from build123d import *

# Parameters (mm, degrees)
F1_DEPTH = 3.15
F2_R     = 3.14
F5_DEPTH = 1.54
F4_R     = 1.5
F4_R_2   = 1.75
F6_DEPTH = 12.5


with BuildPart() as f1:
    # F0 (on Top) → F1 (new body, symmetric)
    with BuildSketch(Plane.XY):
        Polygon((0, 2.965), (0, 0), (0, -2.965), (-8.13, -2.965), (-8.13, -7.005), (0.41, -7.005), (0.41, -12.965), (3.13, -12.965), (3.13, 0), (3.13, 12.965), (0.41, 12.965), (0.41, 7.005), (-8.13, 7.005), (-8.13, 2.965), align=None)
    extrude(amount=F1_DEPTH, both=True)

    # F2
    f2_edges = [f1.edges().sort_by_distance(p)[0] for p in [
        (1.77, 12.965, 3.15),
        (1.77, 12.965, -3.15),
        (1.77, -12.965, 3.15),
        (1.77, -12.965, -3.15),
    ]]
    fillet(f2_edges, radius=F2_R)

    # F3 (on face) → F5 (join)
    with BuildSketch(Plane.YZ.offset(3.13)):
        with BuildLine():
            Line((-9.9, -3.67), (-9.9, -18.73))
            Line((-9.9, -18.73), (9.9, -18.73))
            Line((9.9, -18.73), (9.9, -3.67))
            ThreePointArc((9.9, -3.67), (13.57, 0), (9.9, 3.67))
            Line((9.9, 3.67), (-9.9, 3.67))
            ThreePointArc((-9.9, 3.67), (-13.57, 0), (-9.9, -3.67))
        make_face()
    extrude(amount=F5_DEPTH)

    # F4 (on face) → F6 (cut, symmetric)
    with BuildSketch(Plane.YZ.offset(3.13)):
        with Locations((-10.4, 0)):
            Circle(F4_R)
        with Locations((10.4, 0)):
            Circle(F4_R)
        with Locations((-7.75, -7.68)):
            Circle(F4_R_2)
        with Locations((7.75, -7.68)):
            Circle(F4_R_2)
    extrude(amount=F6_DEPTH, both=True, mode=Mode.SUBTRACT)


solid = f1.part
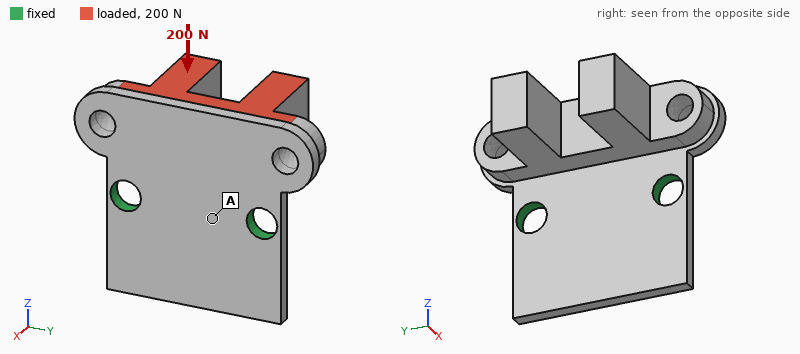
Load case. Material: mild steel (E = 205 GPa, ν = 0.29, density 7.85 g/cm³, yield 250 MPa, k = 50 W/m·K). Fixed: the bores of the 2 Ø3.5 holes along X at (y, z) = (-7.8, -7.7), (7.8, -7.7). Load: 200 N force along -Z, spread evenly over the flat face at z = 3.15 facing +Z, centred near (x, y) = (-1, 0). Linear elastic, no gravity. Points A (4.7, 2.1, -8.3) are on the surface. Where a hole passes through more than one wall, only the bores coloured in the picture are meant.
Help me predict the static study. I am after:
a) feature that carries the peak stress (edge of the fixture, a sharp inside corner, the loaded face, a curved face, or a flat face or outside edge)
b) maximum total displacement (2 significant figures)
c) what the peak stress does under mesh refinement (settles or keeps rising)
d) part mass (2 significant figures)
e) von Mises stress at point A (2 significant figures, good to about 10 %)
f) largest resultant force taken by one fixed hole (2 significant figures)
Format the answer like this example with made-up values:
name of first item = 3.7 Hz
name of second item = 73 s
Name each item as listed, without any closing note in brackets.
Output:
feature that carries the peak stress = edge of the fixture
maximum total displacement = 52 µm
what the peak stress does under mesh refinement = keeps rising
part mass = 12 g
von Mises stress at point A = 29 MPa
largest resultant force taken by one fixed hole = 100 N
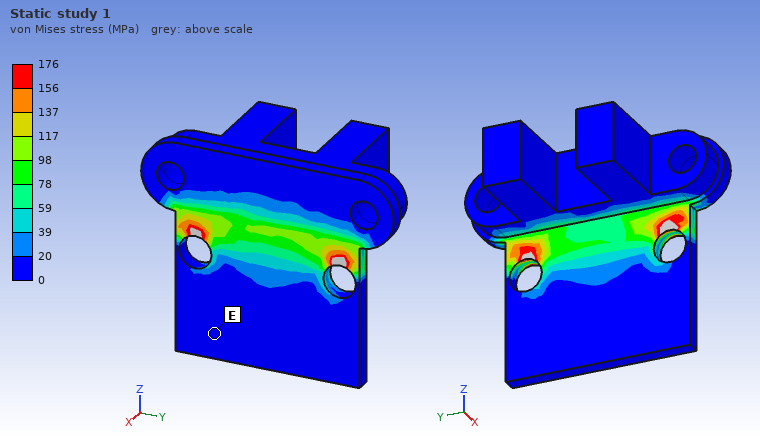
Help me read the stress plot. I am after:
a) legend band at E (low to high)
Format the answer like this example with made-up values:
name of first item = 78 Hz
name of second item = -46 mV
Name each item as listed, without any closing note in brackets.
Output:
legend band at E = 0 to 20 MPa
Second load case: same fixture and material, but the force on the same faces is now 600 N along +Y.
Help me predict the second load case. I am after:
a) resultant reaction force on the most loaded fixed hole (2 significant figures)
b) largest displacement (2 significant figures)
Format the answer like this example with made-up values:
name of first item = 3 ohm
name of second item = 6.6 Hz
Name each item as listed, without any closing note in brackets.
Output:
resultant reaction force on the most loaded fixed hole = 520 N
largest displacement = 15 µm
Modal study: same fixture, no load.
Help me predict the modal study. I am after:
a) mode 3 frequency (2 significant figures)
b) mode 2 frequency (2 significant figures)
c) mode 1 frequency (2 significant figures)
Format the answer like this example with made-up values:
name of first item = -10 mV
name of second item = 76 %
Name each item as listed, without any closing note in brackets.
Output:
mode 3 frequency = 12 kHz
mode 2 frequency = 12 kHz
mode 1 frequency = 4000 Hz
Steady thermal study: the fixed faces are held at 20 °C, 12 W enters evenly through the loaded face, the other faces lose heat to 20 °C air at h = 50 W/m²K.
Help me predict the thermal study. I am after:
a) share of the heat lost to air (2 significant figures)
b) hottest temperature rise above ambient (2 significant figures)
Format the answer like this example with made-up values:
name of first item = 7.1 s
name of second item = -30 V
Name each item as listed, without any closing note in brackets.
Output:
share of the heat lost to air = 17 %
hottest temperature rise above ambient = 57 K
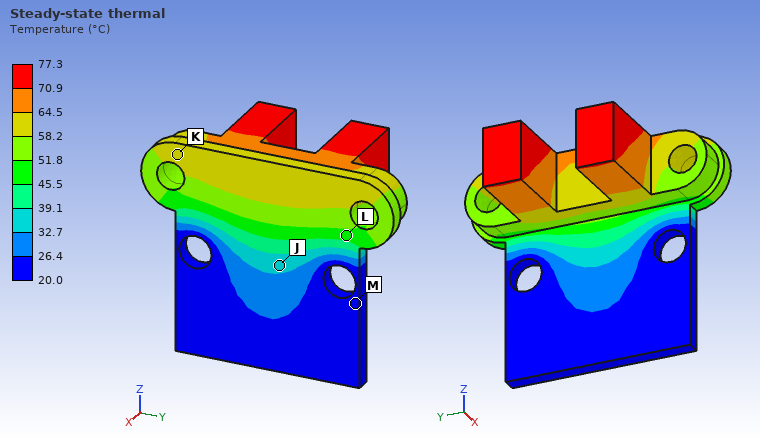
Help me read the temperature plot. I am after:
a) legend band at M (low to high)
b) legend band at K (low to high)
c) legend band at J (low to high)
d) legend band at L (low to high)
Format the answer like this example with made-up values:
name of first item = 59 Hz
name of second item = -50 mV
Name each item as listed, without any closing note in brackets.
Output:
legend band at M = 20.0 to 26.4 °C
legend band at K = 58.2 to 64.5 °C
legend band at J = 32.7 to 39.1 °C
legend band at L = 45.5 to 51.8 °C
